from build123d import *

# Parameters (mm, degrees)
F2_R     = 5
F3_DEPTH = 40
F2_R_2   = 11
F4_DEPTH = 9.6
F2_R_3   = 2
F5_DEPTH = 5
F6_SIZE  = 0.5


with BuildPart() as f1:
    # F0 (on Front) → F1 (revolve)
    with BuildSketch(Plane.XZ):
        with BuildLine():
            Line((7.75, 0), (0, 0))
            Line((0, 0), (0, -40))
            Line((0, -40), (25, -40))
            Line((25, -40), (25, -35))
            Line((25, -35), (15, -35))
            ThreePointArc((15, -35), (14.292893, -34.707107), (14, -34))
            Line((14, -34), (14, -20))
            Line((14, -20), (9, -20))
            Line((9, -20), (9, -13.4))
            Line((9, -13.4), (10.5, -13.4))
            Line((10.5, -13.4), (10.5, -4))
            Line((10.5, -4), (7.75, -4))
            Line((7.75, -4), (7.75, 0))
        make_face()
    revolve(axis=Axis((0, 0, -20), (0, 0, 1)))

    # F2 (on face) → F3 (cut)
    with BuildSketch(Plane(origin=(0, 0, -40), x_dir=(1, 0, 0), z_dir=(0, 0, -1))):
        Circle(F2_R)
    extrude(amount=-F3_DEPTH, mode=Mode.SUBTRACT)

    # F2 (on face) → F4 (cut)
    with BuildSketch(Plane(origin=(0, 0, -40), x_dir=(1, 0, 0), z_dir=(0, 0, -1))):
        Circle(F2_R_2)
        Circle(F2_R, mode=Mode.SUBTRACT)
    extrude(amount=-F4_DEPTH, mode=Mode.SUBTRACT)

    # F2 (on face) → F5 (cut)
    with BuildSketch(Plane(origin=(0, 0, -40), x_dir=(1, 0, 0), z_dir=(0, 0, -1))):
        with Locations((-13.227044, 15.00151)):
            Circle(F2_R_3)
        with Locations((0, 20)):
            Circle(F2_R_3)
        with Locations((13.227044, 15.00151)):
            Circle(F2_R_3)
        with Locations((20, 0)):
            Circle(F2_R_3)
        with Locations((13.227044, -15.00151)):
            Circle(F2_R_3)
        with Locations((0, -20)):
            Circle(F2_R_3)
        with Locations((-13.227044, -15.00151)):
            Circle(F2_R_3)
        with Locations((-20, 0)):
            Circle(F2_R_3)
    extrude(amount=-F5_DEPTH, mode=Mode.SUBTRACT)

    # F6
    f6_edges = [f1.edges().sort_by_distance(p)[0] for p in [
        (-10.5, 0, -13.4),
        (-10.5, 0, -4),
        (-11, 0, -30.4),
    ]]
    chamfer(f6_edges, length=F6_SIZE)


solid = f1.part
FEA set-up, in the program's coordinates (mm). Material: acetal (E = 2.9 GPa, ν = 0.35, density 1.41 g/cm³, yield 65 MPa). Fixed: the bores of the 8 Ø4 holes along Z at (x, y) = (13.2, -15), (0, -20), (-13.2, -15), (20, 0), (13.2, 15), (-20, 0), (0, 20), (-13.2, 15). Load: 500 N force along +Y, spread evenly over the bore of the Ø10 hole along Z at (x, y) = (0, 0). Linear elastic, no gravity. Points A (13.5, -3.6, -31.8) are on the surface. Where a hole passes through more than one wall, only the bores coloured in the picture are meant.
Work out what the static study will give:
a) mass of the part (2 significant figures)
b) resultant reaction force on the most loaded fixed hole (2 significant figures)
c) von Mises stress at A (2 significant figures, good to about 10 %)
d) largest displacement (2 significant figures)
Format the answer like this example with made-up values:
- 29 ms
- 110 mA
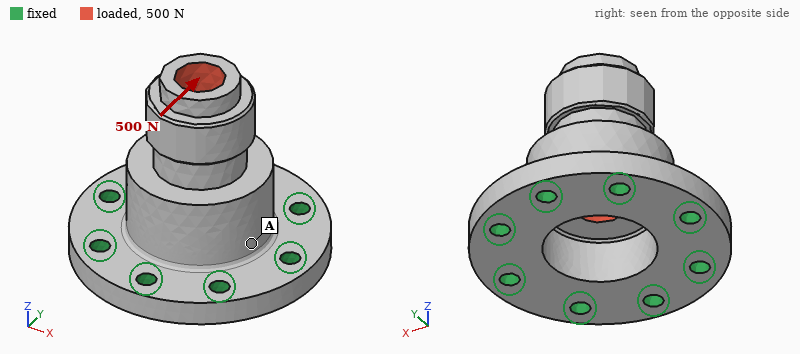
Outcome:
- 26 g
- 190 N
- 2.2 MPa
- 0.21 mm
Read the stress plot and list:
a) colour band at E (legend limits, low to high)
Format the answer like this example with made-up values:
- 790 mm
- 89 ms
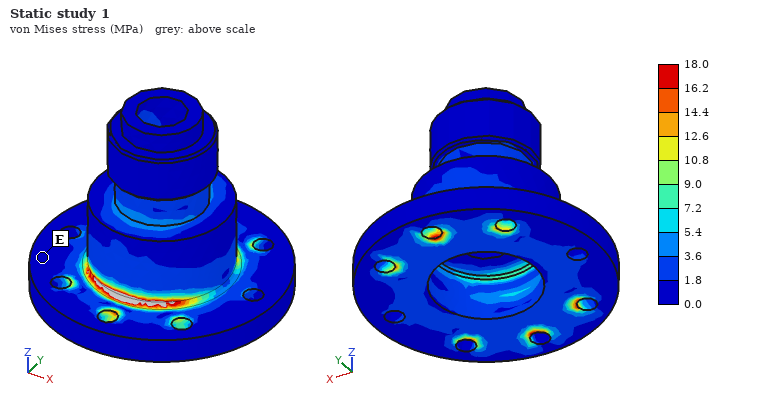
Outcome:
- 0.0 to 1.8 MPa
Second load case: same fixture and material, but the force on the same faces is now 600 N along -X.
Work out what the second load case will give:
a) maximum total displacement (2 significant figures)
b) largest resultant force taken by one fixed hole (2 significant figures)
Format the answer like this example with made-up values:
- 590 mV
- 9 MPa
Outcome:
- 0.25 mm
- 260 N
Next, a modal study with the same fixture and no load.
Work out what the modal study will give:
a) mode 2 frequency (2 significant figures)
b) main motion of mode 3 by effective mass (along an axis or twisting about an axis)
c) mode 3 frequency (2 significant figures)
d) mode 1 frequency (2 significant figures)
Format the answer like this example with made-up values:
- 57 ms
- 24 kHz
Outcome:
- 3000 Hz
- along Z
- 6000 Hz
- 3000 Hz
